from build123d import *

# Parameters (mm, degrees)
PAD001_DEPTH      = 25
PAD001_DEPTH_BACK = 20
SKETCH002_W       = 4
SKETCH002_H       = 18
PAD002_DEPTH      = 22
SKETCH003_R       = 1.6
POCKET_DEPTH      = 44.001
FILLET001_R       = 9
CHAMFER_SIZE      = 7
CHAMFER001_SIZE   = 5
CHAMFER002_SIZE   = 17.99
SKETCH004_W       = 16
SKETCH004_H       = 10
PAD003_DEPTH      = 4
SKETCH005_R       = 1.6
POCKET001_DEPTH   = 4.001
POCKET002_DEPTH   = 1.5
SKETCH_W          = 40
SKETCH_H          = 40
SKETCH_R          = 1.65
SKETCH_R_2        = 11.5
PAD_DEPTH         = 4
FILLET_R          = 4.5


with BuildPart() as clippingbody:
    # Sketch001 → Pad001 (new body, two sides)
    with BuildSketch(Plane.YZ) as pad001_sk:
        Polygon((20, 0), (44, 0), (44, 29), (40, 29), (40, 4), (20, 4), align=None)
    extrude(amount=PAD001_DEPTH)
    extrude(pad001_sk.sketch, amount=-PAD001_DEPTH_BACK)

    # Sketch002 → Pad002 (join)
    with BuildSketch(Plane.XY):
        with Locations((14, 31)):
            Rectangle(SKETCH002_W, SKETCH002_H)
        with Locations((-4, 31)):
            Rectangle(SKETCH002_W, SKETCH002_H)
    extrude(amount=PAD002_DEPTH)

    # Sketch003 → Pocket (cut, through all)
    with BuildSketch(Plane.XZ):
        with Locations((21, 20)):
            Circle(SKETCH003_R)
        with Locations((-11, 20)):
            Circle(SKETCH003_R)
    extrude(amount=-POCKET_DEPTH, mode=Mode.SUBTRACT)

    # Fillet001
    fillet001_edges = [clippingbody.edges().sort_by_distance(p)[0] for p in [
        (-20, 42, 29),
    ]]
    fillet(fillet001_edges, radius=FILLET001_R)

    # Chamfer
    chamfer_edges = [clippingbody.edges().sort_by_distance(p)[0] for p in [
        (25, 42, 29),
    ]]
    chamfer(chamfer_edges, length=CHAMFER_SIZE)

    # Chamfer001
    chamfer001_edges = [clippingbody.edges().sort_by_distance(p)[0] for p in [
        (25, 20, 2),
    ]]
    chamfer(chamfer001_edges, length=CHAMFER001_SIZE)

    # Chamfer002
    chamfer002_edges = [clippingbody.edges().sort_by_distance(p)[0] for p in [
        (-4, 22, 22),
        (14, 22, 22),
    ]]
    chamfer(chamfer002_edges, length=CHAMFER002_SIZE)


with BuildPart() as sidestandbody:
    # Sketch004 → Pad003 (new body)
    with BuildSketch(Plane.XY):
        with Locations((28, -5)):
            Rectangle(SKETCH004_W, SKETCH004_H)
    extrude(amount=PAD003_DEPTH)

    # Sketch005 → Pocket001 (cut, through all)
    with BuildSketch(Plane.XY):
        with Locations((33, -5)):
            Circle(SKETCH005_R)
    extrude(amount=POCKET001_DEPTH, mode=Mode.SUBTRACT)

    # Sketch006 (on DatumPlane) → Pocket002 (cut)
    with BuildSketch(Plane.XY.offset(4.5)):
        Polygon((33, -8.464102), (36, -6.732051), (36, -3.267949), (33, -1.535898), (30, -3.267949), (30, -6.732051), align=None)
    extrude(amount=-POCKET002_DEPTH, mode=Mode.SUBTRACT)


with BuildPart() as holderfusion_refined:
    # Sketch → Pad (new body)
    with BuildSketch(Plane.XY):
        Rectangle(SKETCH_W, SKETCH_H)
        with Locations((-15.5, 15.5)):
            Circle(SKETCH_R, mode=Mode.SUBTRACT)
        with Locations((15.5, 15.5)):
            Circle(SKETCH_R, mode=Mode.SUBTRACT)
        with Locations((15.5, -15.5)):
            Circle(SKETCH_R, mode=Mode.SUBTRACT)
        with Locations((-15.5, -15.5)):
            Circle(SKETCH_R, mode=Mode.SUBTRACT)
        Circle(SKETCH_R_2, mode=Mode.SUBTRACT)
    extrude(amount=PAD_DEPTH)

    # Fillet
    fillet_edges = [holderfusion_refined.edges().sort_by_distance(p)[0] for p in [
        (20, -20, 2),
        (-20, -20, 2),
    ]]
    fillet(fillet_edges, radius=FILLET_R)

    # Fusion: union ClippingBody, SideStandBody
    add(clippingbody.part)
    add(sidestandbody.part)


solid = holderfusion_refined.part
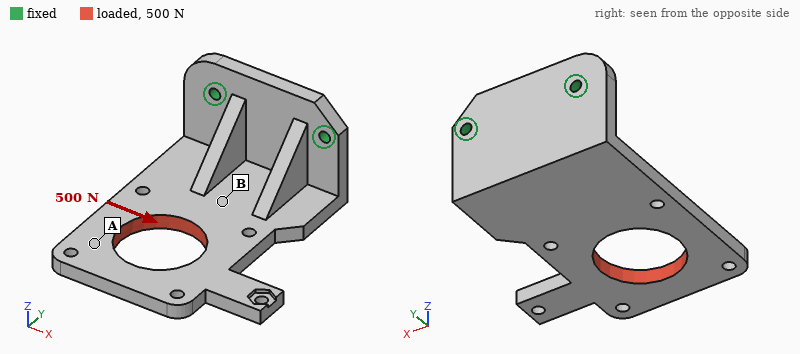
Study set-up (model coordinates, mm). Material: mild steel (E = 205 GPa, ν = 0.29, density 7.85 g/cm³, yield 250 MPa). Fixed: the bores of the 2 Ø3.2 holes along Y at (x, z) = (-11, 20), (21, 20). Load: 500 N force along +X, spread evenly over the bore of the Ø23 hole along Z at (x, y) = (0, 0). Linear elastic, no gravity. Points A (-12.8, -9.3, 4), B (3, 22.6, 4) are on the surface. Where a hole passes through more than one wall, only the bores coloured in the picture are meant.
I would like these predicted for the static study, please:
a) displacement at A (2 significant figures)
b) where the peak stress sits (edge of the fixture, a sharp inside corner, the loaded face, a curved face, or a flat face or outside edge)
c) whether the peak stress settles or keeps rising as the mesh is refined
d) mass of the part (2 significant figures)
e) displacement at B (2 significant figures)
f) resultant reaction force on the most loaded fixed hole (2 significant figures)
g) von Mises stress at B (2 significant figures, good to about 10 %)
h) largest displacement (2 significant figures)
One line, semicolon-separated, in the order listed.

63 µm; edge of the fixture; keeps rising; 120 g; 21 µm; 770 N; 22 MPa; 78 µm
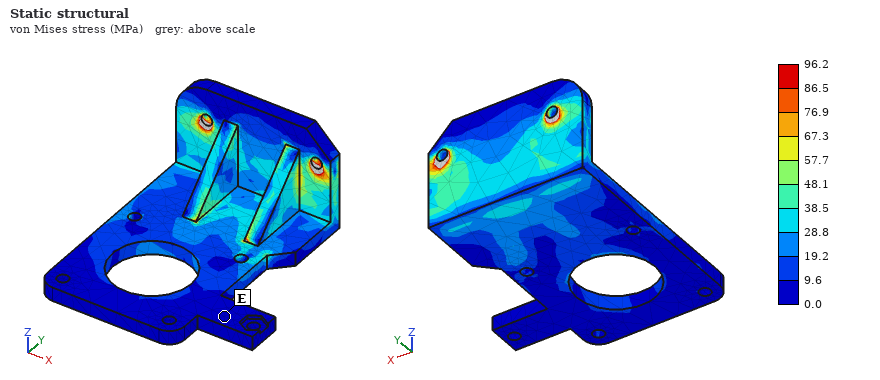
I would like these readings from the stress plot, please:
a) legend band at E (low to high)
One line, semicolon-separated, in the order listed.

0.0 to 9.6 MPa
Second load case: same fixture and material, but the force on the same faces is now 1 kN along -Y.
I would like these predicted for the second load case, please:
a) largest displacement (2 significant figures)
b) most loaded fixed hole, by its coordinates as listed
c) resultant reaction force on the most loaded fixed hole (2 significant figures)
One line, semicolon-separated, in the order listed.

0.15 mm; (-11, 20); 650 N
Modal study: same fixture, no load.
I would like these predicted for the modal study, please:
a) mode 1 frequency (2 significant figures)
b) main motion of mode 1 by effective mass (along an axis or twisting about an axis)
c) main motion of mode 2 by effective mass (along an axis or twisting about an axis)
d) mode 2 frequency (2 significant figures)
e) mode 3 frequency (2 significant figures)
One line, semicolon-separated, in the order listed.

980 Hz; along Z; along X; 2000 Hz; 2600 Hz
